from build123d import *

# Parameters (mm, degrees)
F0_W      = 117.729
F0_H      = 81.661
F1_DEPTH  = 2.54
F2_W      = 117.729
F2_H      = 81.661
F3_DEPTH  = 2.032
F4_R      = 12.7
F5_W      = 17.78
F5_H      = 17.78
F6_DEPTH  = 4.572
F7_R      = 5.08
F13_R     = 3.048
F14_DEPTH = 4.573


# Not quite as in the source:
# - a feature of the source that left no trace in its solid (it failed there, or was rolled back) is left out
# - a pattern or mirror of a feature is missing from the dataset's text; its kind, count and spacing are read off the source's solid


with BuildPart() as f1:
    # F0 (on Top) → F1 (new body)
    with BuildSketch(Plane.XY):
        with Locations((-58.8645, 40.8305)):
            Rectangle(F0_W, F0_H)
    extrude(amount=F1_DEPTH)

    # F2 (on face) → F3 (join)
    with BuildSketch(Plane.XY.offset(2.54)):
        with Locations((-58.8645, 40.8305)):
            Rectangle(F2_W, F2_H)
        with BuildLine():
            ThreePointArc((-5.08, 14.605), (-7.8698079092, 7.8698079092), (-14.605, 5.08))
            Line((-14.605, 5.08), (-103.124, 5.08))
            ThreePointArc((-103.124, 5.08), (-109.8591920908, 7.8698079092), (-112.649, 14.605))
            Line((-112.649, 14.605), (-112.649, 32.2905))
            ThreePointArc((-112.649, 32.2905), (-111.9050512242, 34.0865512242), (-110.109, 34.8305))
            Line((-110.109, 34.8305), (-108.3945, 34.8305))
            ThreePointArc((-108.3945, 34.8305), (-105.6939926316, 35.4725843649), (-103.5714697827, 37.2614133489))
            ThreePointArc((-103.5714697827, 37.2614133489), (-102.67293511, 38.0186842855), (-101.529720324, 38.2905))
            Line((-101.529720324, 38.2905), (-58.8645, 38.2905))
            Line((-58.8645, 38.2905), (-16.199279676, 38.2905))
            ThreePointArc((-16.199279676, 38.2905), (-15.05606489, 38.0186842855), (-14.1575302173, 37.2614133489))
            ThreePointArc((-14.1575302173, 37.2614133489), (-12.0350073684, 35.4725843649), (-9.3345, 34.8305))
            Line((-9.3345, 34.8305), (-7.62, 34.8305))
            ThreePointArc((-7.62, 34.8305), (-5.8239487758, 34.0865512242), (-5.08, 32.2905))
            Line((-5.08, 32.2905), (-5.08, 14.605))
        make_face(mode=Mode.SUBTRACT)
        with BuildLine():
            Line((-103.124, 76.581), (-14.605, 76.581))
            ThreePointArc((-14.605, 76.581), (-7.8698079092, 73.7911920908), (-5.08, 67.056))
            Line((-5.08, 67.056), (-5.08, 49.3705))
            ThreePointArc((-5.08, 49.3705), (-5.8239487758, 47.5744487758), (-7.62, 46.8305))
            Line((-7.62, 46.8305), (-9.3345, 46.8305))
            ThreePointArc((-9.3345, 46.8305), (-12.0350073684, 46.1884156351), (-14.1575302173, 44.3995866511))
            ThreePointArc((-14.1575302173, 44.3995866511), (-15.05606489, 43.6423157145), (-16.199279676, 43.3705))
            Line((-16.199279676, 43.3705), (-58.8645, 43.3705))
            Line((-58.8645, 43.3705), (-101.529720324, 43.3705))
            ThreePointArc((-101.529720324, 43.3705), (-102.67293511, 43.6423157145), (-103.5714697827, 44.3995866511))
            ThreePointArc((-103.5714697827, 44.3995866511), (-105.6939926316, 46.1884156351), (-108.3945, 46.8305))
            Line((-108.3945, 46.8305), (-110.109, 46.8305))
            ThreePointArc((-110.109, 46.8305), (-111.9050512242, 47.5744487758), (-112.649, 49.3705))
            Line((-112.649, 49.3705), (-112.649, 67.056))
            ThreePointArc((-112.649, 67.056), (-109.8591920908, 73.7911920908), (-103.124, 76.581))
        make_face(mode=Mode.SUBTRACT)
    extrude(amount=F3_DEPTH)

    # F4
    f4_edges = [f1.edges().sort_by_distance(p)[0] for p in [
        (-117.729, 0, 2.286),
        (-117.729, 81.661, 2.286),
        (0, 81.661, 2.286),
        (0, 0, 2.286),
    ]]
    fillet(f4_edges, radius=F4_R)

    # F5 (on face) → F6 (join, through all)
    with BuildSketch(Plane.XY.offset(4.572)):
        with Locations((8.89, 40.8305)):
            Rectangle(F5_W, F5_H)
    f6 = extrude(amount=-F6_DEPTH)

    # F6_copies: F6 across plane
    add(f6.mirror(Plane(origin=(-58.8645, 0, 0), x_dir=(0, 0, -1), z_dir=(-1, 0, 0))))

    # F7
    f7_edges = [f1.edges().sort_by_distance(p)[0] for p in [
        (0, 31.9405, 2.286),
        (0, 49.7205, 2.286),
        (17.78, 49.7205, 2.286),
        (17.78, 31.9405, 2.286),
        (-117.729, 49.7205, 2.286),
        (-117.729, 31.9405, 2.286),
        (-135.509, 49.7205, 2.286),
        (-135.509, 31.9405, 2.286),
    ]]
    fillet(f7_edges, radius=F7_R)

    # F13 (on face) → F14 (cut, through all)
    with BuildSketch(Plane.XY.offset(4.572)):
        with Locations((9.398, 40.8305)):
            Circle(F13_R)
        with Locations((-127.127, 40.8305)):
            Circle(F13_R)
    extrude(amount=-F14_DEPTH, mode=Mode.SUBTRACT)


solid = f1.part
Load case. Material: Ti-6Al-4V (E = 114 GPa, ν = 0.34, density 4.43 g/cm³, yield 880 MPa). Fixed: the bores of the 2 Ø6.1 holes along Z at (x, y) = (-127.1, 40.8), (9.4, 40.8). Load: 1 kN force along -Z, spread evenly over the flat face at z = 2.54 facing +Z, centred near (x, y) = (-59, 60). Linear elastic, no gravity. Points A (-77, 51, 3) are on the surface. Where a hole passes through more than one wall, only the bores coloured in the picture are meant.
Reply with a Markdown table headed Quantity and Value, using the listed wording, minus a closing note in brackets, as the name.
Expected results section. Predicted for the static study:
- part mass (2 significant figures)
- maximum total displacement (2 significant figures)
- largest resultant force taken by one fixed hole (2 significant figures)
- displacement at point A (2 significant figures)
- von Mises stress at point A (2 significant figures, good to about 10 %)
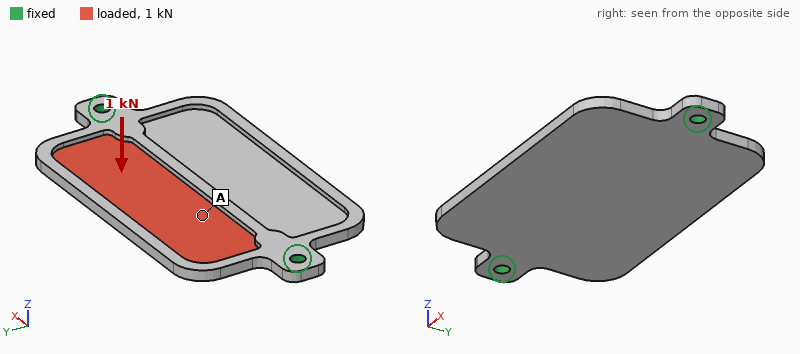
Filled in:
| Quantity | Value |
|---|---|
| part mass | 140 g |
| maximum total displacement | 0.91 mm |
| largest resultant force taken by one fixed hole | 1.1 kN |
| displacement at point A | 0.42 mm |
| von Mises stress at point A | 35 MPa |
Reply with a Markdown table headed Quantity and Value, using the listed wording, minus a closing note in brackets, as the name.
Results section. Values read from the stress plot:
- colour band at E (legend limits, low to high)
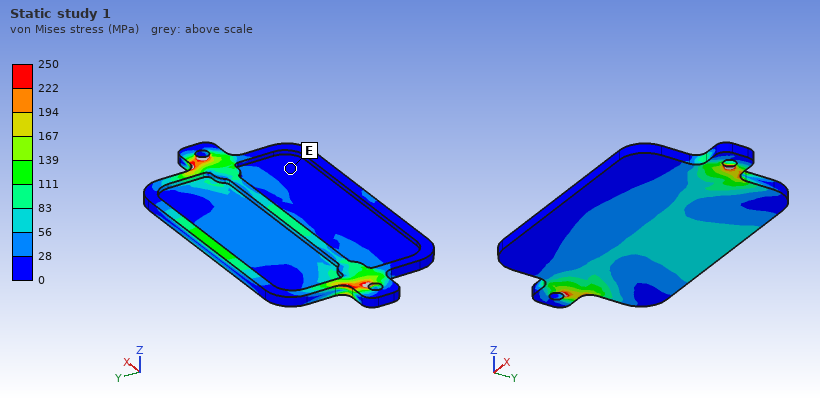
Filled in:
| Quantity | Value |
|---|---|
| colour band at E | 0 to 28 MPa |
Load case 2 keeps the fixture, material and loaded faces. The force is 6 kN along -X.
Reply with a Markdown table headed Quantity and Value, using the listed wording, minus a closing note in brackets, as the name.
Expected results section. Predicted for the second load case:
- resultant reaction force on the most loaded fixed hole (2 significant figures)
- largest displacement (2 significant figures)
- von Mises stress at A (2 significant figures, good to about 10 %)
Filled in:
| Quantity | Value |
|---|---|
| resultant reaction force on the most loaded fixed hole | 3.1 kN |
| largest displacement | 67 µm |
| von Mises stress at A | 27 MPa |
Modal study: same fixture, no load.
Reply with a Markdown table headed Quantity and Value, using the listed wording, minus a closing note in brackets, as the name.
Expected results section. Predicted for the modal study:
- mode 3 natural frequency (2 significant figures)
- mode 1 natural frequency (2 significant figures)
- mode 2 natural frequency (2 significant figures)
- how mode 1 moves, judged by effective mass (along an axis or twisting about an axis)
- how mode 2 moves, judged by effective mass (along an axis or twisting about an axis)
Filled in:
| Quantity | Value |
|---|---|
| mode 3 natural frequency | 1800 Hz |
| mode 1 natural frequency | 790 Hz |
| mode 2 natural frequency | 860 Hz |
| how mode 1 moves, judged by effective mass | twisting about X |
| how mode 2 moves, judged by effective mass | along Z |
